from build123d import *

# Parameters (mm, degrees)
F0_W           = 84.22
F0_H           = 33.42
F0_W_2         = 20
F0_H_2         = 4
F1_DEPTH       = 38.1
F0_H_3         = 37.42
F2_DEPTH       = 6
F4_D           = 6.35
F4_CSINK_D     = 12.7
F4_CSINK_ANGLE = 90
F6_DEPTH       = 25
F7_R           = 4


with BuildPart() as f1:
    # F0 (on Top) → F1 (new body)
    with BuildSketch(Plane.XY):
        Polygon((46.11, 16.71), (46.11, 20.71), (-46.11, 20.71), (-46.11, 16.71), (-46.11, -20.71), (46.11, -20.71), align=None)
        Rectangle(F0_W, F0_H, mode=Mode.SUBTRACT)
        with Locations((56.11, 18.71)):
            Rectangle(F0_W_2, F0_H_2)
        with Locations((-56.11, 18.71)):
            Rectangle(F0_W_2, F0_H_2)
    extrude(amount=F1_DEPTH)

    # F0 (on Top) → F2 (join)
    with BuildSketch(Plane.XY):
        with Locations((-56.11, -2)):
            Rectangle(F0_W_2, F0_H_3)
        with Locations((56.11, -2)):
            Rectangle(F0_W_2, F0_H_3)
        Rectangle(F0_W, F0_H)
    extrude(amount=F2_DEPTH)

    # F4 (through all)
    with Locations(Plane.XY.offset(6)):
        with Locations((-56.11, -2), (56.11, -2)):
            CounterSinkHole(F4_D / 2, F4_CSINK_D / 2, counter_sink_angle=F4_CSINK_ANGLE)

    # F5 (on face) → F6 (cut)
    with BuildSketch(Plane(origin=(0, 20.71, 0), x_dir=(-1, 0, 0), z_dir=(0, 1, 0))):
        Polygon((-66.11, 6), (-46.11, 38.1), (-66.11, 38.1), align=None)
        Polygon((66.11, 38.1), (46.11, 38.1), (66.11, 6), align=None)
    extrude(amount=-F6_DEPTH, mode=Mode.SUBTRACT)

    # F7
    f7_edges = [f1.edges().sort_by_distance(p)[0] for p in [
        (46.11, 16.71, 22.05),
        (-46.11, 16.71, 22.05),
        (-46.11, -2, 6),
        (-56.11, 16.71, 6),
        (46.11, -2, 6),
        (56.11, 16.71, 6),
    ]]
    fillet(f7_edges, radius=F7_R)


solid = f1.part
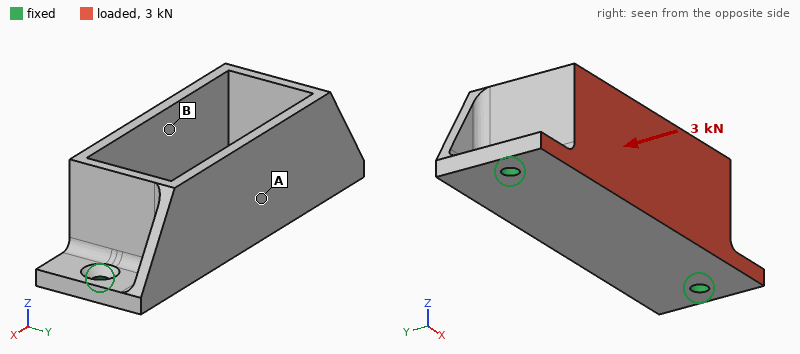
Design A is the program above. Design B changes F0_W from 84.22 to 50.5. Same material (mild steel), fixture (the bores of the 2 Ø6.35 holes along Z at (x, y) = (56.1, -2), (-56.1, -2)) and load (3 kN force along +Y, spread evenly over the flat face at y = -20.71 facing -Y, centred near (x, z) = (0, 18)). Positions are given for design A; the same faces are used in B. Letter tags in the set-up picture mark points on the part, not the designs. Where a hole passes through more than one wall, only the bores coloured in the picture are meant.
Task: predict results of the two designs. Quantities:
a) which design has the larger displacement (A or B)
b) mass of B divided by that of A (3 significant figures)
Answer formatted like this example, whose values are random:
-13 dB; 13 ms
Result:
A; 1.53
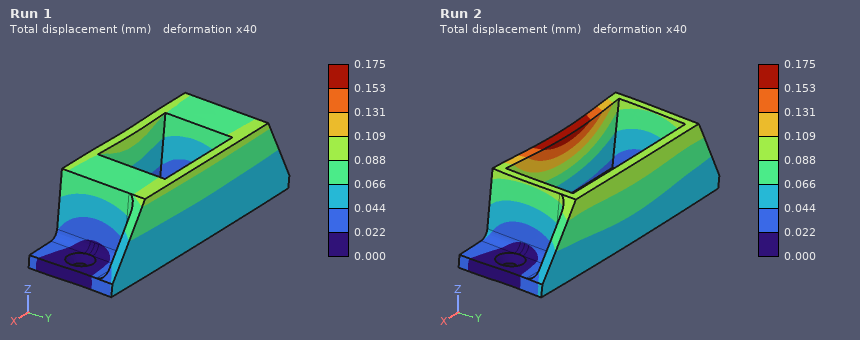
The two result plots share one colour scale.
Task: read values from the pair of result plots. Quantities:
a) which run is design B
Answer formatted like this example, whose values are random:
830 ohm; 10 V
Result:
Run 1
